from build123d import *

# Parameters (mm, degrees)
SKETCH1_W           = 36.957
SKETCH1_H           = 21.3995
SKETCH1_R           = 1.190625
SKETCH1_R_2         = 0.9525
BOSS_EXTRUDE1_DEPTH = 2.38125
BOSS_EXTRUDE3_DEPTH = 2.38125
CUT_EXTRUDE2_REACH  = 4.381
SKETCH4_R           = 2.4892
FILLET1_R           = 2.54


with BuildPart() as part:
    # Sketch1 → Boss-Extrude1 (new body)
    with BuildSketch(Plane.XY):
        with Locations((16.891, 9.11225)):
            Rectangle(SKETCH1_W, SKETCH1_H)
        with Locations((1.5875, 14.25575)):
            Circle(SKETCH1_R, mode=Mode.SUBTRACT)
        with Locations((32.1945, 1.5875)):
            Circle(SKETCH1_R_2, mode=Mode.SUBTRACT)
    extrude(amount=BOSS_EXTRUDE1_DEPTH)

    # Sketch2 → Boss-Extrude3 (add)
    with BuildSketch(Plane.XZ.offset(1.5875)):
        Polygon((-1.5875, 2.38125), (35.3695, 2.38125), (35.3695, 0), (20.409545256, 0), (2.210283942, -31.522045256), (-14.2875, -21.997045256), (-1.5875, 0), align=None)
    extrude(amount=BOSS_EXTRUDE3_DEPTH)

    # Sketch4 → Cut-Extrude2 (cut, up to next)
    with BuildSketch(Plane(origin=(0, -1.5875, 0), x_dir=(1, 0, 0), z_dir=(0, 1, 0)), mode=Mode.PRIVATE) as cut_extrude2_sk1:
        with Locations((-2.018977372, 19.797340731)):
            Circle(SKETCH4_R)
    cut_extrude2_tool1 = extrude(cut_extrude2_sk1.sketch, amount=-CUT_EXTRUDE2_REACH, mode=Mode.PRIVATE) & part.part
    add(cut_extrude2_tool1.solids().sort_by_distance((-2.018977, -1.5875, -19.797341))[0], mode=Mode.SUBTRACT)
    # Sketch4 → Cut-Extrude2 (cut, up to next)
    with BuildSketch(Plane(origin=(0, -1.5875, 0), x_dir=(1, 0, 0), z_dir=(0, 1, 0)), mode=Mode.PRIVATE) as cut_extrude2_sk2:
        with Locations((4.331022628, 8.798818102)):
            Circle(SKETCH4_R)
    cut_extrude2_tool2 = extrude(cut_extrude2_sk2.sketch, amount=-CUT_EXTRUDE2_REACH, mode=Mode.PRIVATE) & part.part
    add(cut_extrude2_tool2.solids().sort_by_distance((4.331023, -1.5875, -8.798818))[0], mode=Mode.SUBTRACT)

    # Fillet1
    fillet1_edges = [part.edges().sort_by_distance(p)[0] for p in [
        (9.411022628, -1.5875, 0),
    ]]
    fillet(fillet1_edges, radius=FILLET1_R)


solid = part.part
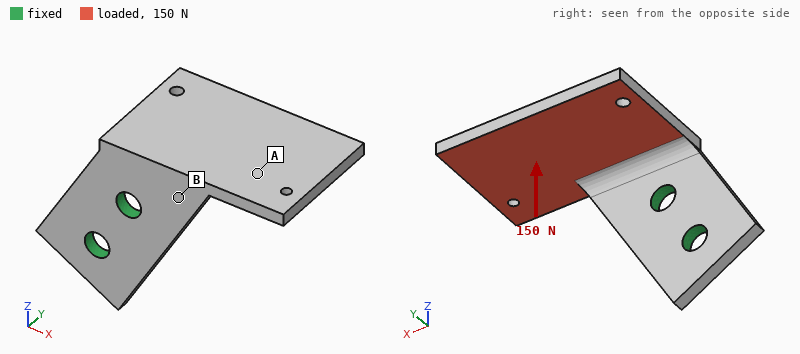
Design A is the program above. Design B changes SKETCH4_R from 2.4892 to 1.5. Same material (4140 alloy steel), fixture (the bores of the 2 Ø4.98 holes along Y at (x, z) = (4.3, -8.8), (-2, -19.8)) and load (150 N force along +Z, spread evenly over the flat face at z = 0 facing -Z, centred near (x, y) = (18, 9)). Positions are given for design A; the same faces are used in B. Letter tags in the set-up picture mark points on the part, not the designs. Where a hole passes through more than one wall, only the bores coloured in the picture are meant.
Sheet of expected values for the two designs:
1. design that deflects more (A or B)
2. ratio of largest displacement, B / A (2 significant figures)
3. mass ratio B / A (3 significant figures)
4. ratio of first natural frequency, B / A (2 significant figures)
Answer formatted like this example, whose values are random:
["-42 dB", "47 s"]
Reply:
["B", "1.1", "1.02", "0.91"]
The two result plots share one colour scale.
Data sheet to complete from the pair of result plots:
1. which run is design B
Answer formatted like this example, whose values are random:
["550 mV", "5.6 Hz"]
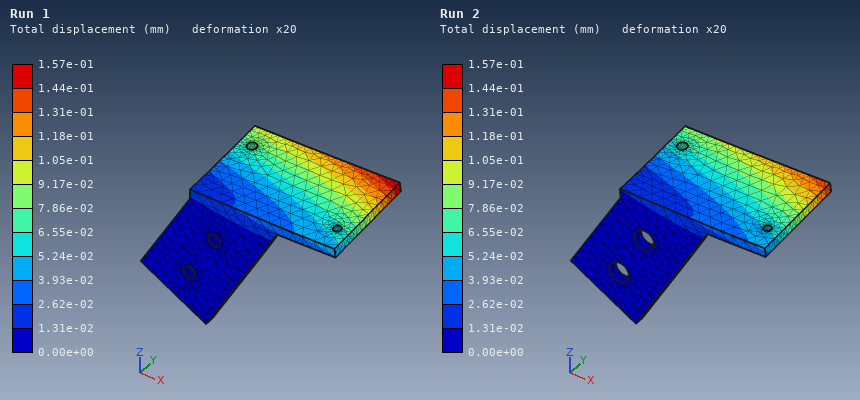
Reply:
["Run 1"]
